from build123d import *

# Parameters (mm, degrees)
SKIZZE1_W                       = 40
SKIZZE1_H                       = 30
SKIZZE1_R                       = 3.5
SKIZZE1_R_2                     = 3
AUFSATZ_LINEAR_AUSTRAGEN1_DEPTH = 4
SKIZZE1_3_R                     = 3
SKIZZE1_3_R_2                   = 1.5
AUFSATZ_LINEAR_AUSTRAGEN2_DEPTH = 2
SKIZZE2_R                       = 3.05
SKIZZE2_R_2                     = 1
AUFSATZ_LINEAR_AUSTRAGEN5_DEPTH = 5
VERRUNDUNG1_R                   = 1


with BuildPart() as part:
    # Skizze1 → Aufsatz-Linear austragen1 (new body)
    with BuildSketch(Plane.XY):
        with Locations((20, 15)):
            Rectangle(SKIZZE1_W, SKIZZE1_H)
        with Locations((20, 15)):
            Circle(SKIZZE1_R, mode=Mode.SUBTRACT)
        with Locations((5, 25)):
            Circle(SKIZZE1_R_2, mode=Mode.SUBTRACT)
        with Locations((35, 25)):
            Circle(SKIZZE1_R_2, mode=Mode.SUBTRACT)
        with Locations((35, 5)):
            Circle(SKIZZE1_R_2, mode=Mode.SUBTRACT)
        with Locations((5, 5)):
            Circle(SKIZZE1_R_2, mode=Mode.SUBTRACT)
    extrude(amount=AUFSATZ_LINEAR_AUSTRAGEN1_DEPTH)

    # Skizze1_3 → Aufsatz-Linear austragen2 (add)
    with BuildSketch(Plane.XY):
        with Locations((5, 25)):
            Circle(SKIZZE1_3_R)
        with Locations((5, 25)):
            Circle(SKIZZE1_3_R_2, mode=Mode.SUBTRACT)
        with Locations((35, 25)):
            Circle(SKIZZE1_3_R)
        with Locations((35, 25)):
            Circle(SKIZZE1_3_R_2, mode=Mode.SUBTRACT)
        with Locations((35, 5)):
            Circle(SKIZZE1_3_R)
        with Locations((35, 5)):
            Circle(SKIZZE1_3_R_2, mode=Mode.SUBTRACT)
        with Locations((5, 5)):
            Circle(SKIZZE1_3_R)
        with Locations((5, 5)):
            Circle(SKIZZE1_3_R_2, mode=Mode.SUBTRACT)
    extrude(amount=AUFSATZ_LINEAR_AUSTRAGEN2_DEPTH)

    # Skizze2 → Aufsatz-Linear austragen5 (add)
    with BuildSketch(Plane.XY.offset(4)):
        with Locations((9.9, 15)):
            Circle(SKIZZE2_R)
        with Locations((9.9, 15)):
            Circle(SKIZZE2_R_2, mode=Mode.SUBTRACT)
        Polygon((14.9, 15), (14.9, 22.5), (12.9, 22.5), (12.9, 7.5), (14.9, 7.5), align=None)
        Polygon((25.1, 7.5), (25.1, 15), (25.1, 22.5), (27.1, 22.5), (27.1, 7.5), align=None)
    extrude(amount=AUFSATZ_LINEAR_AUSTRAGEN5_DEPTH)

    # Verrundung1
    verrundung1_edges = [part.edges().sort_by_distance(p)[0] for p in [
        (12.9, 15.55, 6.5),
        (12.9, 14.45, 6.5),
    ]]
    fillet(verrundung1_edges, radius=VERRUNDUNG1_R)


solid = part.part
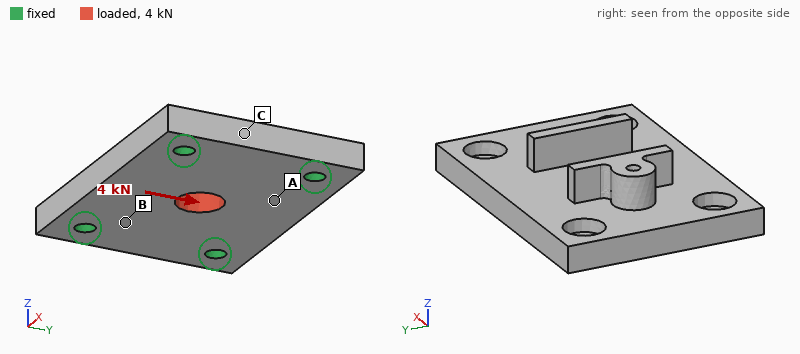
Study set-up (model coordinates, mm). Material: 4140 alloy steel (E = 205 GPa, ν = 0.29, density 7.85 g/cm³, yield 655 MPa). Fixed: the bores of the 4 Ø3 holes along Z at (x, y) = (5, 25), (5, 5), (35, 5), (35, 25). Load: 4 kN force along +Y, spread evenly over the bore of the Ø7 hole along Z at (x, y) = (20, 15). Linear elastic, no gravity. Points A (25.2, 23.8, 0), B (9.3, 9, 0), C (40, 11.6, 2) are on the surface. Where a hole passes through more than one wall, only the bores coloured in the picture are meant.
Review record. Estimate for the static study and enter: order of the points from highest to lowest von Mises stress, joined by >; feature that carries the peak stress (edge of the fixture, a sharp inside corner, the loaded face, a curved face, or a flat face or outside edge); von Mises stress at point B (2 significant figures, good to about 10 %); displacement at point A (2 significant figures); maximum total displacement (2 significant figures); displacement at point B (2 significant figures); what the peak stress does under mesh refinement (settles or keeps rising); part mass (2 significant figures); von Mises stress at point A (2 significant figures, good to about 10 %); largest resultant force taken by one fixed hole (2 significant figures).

B > A > C
edge of the fixture
49 MPa
3.3 µm
4.8 µm
1.8 µm
keeps rising
38 g
31 MPa
1.1 kN
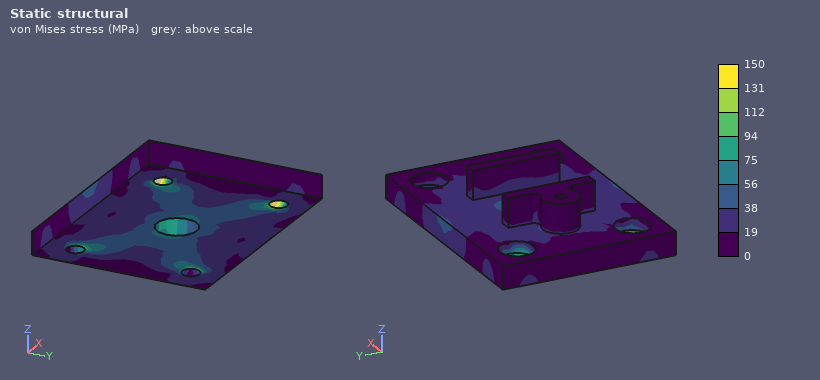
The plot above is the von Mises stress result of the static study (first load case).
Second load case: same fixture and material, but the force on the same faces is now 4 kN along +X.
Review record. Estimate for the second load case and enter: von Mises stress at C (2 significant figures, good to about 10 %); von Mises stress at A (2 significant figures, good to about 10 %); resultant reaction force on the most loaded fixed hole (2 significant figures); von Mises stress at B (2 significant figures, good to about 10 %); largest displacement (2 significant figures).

17 MPa
24 MPa
1.0 kN
41 MPa
3.2 µm
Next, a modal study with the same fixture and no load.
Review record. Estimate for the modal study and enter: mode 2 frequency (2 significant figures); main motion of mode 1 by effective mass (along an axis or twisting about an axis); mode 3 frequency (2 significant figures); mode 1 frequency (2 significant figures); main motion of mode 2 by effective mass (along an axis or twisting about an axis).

20 kHz
along Z
31 kHz
14 kHz
twisting about X
